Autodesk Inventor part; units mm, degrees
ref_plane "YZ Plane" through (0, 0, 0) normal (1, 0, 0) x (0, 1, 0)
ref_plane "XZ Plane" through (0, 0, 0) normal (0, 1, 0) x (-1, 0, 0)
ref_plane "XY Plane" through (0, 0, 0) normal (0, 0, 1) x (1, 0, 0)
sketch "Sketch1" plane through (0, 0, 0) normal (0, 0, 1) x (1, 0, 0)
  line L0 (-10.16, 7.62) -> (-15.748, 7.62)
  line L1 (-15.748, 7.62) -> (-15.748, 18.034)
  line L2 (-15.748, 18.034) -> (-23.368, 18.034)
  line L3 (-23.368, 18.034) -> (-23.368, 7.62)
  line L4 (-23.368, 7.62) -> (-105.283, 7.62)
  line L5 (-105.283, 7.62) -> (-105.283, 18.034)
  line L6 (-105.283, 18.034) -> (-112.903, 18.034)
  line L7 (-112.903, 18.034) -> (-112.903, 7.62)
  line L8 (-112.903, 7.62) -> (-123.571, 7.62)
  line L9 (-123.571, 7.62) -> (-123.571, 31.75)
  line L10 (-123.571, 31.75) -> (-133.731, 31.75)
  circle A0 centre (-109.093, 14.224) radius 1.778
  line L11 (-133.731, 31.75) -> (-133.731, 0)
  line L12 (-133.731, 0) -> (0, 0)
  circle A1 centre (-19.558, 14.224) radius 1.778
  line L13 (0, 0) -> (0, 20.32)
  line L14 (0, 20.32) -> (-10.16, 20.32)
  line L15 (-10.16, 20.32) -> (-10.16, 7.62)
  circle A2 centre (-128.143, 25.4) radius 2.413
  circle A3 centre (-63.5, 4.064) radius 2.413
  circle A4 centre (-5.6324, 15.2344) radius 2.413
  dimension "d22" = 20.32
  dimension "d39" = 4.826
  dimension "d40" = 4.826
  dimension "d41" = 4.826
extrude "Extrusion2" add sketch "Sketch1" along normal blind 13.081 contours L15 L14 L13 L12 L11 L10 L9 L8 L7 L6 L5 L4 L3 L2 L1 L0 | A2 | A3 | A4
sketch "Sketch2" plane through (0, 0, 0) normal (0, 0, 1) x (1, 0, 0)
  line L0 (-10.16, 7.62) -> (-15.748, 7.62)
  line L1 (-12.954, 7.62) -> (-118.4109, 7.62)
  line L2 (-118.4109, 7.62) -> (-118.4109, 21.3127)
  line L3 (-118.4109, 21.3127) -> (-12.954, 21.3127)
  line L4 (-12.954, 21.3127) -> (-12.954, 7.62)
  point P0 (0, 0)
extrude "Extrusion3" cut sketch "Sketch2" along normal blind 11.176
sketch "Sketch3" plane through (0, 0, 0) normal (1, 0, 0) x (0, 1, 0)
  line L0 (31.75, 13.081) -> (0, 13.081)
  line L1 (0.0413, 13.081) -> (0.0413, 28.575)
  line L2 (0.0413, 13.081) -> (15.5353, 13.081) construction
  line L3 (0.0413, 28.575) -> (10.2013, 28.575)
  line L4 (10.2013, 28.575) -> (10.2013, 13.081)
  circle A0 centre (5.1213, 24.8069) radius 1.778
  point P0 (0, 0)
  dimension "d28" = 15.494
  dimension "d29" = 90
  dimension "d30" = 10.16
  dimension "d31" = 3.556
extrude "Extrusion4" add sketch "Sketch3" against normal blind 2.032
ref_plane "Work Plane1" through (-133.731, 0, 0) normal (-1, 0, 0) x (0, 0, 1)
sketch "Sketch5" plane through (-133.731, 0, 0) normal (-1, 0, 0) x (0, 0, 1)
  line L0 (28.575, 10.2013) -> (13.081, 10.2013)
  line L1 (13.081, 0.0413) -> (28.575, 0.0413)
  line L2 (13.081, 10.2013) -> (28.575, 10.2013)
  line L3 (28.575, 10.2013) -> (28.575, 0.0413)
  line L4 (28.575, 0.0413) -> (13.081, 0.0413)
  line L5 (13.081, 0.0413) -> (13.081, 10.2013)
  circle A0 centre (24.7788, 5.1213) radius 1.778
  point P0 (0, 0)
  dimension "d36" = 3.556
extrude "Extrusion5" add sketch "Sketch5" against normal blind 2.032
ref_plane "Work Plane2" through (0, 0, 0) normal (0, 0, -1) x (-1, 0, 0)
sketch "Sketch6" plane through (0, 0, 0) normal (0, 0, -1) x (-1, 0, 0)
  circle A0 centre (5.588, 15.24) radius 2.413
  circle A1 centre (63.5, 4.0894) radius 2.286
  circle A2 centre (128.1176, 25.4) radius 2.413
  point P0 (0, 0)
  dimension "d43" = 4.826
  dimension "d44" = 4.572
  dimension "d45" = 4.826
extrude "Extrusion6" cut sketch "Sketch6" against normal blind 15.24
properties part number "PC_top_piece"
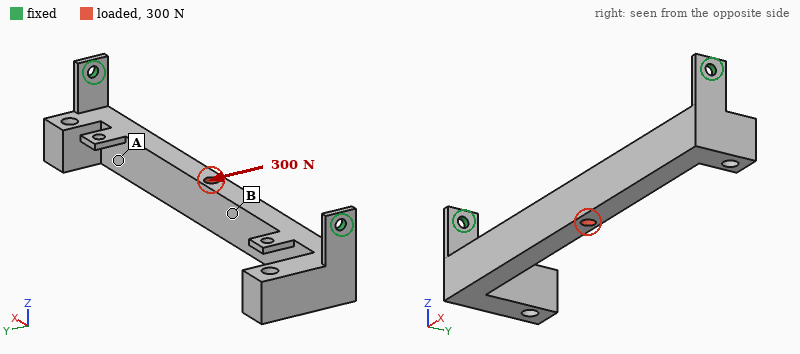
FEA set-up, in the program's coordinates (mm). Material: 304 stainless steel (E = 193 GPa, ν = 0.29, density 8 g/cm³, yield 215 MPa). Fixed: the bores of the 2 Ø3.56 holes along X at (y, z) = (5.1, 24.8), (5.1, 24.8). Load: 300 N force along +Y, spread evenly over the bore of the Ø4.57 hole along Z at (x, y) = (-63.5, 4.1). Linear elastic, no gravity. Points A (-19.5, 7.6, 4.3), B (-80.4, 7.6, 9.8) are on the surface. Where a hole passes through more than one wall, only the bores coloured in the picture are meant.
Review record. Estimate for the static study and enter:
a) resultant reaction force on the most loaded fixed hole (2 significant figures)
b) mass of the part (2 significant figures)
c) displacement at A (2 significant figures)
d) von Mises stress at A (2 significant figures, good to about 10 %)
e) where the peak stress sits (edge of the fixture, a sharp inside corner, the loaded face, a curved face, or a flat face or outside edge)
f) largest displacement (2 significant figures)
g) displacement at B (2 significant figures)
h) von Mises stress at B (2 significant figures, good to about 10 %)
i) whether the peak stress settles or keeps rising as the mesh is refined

160 N
150 g
0.076 mm
17 MPa
edge of the fixture
0.16 mm
0.14 mm
52 MPa
keeps rising
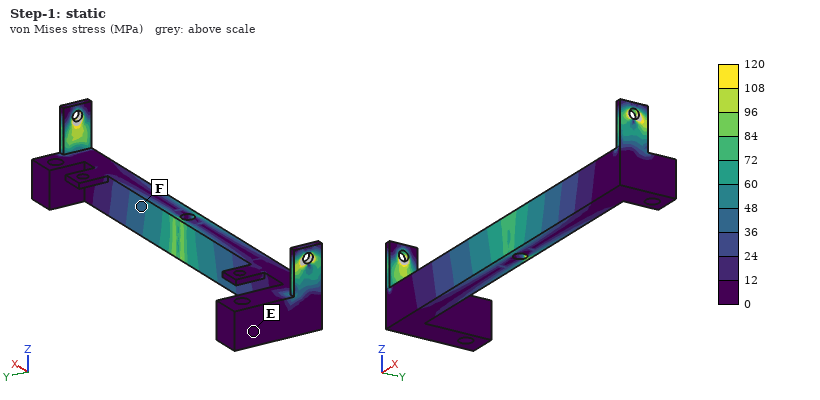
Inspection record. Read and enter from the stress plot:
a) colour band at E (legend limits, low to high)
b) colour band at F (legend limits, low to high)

0 to 12 MPa
36 to 48 MPa
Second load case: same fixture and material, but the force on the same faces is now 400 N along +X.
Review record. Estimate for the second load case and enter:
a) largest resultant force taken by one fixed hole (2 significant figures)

200 N
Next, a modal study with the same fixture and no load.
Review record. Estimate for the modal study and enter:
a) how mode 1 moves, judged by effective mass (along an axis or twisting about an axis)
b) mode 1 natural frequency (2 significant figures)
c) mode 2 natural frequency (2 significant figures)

along Y
900 Hz
1700 Hz
